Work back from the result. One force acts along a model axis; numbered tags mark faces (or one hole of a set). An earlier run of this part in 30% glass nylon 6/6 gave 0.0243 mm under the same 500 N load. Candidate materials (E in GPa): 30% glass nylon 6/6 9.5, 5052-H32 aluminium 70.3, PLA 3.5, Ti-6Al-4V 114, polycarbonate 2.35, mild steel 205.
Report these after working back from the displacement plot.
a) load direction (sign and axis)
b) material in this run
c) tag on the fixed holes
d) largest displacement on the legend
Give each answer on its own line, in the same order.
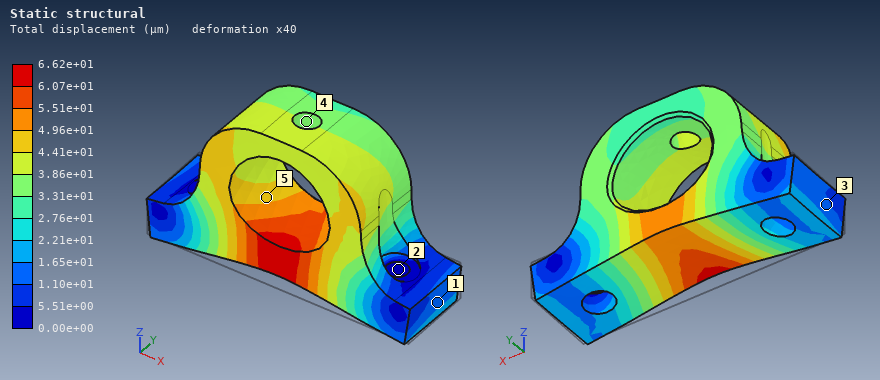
+Z
PLA
2
6.62e+01 µm
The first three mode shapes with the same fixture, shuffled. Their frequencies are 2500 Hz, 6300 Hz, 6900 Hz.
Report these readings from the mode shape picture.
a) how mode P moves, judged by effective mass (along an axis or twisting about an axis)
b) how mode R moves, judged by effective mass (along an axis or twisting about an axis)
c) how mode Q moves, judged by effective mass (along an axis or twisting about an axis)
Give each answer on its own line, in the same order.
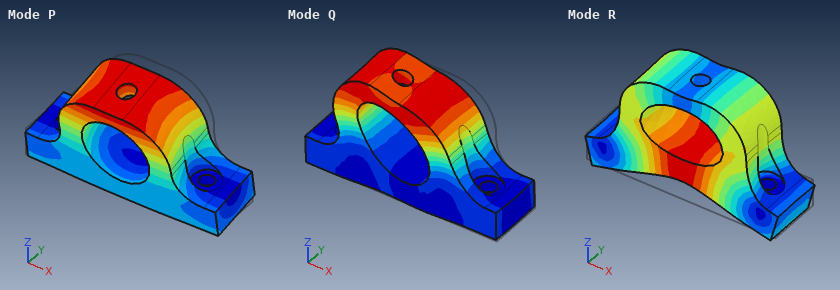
along Y
along Z
along X
